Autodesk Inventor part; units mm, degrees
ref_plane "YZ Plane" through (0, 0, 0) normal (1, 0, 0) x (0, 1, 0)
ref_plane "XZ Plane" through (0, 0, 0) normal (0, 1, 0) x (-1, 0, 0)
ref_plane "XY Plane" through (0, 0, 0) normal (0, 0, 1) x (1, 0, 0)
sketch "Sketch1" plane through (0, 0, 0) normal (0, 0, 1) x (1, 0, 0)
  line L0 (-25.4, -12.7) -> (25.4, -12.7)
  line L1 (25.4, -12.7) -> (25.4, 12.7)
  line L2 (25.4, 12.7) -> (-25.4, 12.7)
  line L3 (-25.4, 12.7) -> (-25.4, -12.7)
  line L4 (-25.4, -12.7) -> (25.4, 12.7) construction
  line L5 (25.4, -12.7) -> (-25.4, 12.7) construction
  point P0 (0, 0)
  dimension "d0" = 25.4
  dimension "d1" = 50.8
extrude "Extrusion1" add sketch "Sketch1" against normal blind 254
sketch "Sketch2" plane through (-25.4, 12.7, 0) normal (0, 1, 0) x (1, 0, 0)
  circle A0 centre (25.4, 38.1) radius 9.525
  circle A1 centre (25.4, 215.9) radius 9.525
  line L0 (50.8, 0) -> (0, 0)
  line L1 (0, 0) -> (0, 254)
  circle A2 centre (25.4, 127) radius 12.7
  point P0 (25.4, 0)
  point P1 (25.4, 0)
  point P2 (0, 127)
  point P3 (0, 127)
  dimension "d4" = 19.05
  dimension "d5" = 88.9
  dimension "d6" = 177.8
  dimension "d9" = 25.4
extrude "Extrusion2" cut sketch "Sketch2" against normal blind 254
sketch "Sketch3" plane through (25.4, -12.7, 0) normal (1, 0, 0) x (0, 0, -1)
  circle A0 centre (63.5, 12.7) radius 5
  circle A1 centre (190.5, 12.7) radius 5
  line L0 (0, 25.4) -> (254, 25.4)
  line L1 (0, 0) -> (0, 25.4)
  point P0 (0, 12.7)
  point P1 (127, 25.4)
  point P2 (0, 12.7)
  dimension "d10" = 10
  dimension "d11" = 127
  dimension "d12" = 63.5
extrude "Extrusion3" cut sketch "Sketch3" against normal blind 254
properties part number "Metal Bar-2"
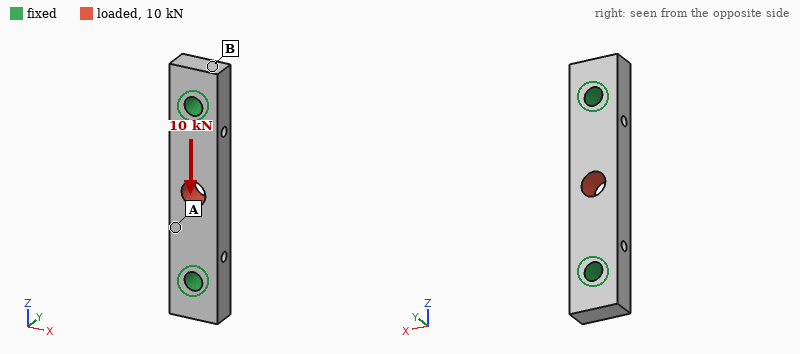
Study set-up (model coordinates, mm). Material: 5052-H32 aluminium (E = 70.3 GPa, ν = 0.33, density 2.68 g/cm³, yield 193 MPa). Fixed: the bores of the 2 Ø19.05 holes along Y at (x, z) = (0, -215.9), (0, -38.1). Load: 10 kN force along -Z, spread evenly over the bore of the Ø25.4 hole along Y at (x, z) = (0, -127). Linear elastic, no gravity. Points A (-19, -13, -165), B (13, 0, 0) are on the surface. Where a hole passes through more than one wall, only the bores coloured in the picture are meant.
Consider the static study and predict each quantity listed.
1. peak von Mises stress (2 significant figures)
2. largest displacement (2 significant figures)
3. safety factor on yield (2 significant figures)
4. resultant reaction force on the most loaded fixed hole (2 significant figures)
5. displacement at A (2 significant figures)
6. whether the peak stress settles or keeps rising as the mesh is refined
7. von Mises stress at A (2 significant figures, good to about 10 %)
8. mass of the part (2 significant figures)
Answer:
15 MPa
5.7 µm
13
5.0 kN
3.5 µm
settles
3.8 MPa
780 g
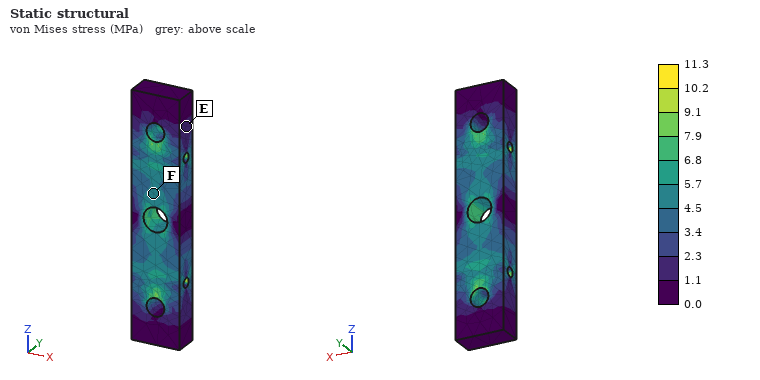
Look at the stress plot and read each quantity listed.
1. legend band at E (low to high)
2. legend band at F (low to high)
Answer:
1.1 to 2.3 MPa
4.5 to 5.7 MPa
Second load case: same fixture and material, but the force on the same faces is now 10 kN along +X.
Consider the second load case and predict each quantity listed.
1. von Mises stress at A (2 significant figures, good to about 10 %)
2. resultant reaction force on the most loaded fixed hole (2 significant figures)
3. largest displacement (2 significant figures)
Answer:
6.7 MPa
5.0 kN
36 µm
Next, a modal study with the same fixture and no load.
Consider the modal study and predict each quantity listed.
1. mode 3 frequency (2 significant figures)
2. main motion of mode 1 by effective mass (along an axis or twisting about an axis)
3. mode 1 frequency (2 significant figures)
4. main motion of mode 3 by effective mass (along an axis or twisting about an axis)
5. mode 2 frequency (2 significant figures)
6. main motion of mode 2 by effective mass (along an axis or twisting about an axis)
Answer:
6800 Hz
along Y
3900 Hz
twisting about Z
5500 Hz
along X
